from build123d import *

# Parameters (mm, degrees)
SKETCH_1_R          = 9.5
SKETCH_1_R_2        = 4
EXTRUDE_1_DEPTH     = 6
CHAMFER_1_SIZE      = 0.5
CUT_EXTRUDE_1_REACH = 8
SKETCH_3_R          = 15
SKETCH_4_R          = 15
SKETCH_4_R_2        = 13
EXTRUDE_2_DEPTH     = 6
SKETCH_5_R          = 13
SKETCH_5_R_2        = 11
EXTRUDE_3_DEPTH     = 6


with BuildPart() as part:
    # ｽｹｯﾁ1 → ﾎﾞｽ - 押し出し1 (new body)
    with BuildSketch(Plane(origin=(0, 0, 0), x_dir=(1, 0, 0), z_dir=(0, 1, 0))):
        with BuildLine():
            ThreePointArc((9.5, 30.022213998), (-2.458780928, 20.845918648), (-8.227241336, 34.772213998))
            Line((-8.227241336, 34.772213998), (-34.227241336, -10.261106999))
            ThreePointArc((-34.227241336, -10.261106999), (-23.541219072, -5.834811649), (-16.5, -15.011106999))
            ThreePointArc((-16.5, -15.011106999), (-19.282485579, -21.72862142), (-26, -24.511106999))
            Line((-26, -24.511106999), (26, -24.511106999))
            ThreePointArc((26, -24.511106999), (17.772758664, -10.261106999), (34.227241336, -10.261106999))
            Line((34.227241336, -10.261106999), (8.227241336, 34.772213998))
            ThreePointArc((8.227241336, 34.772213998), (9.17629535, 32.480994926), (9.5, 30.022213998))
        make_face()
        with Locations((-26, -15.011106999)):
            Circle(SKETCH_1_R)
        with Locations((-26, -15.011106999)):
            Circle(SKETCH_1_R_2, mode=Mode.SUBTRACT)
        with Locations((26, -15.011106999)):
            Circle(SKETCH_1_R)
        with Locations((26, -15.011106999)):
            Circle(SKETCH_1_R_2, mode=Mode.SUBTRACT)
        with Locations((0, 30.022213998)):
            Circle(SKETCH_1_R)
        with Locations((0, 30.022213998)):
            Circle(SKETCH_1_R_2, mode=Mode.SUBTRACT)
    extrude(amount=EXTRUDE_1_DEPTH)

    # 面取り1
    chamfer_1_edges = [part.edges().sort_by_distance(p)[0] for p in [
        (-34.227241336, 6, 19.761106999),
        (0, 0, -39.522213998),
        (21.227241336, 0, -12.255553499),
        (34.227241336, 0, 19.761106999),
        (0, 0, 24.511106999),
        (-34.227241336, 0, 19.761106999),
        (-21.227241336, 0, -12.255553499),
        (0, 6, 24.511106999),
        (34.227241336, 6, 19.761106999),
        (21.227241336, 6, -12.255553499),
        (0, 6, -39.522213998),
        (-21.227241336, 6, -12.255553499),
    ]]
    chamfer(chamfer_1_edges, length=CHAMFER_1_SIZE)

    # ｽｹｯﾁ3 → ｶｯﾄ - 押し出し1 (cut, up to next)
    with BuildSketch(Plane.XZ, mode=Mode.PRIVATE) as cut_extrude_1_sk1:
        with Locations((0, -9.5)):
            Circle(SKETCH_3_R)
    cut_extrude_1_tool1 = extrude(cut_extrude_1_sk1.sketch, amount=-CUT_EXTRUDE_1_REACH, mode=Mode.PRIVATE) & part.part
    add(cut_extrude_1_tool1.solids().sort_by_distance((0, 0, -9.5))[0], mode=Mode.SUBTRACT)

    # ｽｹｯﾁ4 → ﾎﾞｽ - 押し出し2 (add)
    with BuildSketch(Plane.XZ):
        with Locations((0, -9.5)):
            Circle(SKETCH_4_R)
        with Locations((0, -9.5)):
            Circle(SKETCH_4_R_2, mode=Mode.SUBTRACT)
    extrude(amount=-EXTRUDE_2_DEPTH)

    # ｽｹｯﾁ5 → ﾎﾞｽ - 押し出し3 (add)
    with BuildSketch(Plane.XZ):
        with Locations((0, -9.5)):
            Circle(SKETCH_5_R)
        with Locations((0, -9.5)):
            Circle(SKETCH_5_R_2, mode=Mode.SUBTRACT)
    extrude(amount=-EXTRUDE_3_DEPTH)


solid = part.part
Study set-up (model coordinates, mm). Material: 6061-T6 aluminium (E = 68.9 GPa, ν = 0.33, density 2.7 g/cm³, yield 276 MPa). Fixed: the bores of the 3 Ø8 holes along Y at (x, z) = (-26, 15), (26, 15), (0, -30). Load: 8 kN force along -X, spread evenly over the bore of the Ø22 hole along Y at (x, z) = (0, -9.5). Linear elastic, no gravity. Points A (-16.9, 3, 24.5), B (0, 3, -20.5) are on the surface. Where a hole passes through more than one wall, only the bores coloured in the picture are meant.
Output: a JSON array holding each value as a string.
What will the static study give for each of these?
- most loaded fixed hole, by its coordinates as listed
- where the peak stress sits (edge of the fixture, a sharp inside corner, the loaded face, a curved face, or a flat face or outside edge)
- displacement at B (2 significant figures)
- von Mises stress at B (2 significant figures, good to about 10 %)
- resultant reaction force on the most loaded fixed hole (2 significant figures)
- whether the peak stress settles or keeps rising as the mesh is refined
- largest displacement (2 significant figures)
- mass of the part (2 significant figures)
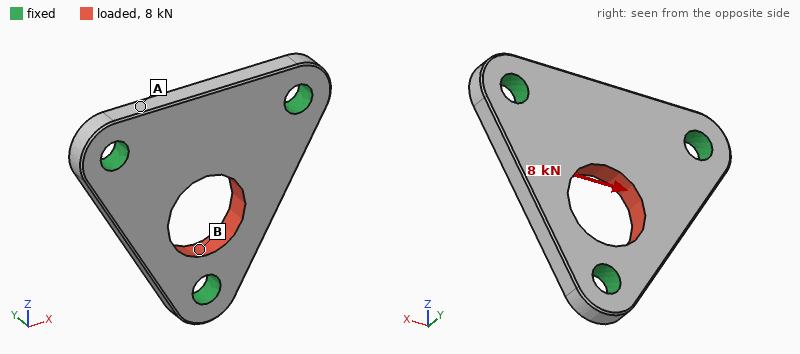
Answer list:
["(0, -30)", "edge of the fixture", "9.4 µm", "37 MPa", "3.6 kN", "keeps rising", "17 µm", "39 g"]
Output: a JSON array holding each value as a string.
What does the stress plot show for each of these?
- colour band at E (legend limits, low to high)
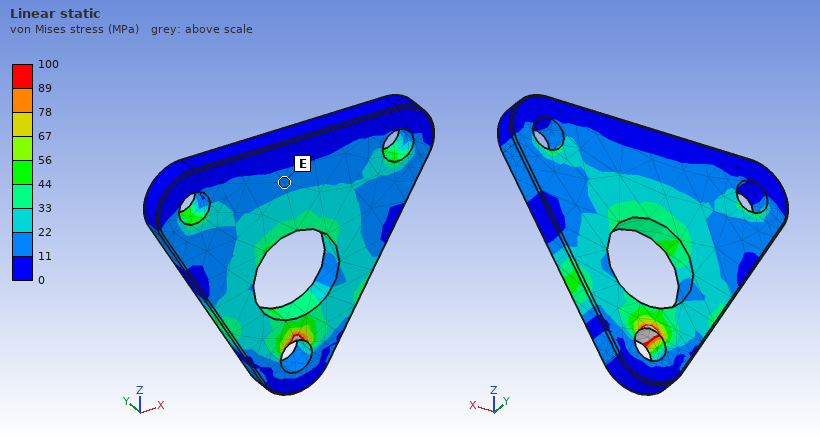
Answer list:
["11 to 22 MPa"]
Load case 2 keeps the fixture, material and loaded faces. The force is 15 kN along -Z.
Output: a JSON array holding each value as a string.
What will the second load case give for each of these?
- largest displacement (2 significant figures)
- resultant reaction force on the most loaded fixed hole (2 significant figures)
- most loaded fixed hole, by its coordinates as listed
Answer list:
["32 µm", "6.0 kN", "(0, -30)"]
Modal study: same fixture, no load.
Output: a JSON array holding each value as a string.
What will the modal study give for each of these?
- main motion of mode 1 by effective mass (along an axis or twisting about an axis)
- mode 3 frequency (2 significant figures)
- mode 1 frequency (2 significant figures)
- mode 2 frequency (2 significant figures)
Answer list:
["along Y", "14 kHz", "12 kHz", "14 kHz"]
